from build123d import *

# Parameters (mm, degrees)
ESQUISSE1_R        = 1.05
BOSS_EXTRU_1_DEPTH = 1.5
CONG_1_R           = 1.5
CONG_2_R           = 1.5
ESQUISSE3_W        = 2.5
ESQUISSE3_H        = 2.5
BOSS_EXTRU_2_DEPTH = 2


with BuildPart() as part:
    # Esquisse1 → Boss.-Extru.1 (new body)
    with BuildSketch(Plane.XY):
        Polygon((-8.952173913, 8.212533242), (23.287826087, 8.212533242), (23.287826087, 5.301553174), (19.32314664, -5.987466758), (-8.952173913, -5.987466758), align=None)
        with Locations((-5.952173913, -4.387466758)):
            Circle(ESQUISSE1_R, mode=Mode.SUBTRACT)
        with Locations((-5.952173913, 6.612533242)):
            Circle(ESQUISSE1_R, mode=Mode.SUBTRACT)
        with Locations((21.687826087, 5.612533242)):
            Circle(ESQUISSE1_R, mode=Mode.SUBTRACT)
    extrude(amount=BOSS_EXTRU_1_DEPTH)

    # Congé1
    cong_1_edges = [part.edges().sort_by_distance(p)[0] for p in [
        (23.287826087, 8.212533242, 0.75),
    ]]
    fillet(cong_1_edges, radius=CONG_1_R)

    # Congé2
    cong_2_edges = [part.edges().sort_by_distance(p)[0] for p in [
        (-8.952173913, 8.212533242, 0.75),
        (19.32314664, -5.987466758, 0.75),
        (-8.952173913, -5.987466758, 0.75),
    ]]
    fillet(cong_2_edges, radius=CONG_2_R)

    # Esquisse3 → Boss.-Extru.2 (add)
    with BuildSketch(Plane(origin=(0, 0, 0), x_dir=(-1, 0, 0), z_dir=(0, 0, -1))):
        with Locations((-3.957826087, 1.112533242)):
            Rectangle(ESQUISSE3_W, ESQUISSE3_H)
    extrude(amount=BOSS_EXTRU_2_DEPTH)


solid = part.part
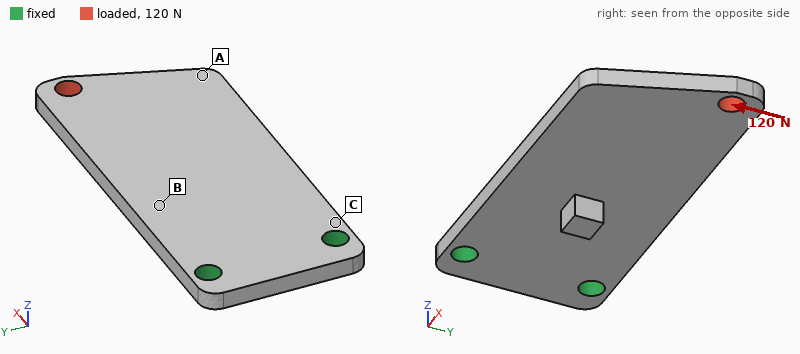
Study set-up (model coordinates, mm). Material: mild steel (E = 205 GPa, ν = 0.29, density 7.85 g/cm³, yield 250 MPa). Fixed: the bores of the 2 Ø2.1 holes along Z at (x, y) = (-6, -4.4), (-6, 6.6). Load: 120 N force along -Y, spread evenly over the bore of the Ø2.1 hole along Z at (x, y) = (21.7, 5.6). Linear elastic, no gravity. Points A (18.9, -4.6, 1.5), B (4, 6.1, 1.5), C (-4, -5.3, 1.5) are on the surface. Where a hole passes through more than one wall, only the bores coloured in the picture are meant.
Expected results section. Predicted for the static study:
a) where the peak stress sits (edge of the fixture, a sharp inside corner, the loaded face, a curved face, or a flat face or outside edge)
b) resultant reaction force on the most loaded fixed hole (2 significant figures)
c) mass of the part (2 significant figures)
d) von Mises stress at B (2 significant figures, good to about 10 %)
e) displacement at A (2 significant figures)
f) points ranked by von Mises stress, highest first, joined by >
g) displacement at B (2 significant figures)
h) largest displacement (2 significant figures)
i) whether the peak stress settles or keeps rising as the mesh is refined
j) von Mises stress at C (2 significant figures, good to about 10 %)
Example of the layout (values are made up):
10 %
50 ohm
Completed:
edge of the fixture
300 N
5.1 g
30 MPa
12 µm
C > B > A
3.1 µm
16 µm
keeps rising
57 MPa
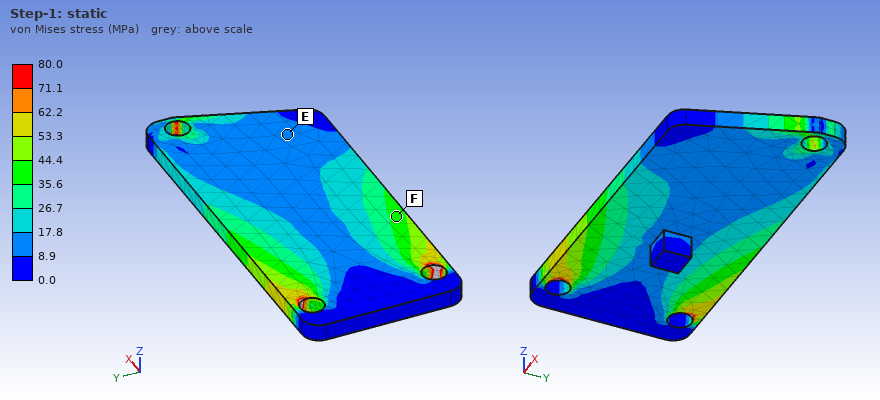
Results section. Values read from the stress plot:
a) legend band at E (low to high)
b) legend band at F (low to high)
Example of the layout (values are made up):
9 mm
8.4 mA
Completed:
8.9 to 17.8 MPa
35.6 to 44.4 MPa
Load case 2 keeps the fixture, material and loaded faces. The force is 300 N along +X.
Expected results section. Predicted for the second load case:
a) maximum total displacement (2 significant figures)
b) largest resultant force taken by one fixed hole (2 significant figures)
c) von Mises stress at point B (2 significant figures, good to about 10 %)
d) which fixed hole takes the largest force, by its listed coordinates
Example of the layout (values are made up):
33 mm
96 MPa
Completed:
9.8 µm
270 N
34 MPa
(-6, 6.6)
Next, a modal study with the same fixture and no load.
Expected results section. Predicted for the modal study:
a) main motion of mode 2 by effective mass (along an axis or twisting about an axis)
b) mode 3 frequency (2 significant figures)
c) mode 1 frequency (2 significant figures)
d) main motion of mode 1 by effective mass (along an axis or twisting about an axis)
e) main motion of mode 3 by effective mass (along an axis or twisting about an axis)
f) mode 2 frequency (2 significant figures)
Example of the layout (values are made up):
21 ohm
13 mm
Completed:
twisting about X
10 kHz
1700 Hz
along Z
along Z
7200 Hz
